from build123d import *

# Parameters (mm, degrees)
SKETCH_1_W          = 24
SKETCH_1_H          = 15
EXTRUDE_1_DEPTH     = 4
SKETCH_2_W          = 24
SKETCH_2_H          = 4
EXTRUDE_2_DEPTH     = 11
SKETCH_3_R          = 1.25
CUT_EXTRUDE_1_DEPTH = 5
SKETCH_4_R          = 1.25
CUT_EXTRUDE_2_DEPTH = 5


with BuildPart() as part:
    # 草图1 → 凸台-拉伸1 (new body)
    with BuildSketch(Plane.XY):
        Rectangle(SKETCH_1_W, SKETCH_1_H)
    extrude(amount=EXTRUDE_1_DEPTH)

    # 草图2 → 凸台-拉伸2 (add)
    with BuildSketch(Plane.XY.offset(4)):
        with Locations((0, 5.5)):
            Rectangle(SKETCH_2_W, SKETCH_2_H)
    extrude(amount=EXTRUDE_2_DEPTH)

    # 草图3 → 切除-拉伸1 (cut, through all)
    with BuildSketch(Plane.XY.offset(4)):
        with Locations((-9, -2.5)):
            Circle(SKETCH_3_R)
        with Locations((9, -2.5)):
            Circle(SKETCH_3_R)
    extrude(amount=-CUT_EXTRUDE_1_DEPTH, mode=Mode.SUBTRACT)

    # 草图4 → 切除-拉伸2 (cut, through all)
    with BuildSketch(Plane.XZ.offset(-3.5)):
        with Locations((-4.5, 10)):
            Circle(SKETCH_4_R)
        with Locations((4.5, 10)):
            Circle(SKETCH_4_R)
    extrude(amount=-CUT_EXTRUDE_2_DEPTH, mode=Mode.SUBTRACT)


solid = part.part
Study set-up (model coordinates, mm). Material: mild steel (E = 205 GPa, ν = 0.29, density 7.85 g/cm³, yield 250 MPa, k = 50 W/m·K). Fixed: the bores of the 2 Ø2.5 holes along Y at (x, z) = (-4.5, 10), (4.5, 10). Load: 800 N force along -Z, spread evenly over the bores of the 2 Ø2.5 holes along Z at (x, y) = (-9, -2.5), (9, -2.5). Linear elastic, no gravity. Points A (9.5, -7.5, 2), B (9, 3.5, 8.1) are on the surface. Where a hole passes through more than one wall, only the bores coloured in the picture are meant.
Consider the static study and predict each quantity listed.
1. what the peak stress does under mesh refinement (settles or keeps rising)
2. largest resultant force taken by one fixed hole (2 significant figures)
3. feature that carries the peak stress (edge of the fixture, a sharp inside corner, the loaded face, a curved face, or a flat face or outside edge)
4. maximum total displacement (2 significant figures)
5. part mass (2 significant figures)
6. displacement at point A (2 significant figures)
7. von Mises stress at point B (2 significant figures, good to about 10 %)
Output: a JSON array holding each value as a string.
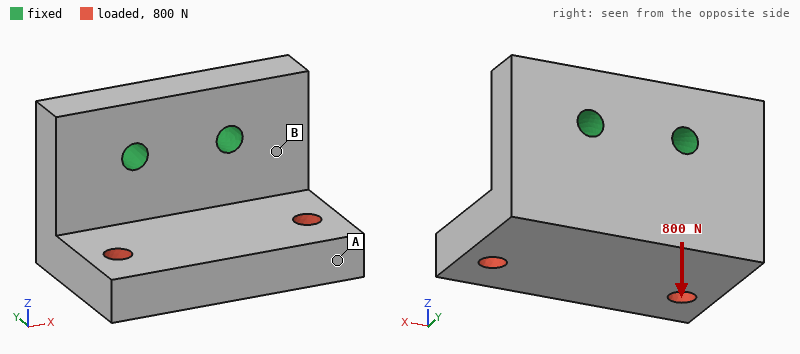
["keeps rising", "400 N", "edge of the fixture", "37 µm", "19 g", "34 µm", "74 MPa"]
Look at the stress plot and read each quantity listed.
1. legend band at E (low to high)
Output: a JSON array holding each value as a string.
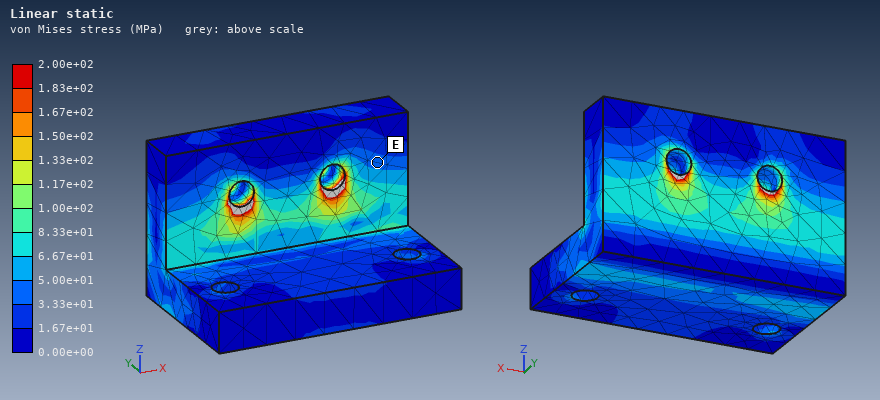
["3.33e+01 to 5.00e+01 MPa"]
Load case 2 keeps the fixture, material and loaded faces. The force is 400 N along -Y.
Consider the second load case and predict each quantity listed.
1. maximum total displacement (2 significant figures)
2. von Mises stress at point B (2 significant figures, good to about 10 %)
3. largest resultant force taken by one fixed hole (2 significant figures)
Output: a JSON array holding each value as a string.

["8.7 µm", "22 MPa", "200 N"]
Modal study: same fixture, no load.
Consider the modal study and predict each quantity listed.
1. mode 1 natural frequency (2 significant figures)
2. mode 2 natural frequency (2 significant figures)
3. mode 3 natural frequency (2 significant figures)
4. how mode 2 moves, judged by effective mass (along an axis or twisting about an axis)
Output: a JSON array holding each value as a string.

["9500 Hz", "14 kHz", "23 kHz", "along X"]
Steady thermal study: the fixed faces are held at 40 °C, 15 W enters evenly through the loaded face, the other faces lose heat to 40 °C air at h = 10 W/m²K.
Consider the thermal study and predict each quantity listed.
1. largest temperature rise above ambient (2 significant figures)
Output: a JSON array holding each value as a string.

["57 K"]
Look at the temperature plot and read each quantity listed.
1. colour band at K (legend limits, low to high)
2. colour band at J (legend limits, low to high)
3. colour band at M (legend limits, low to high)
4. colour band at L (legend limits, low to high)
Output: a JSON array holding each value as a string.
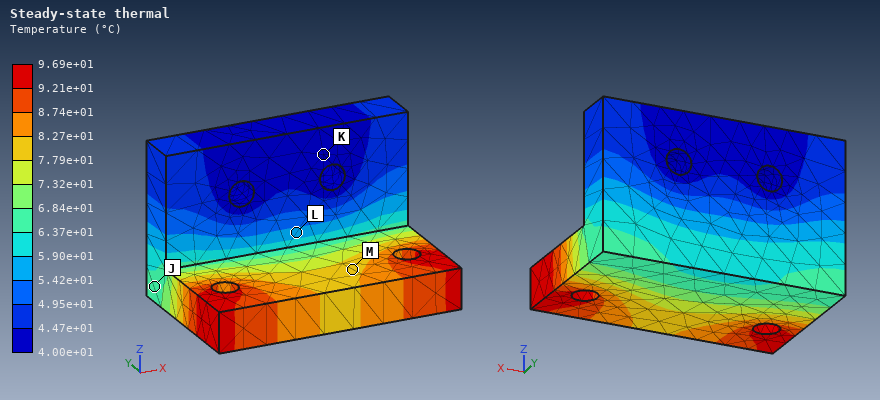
["4.00e+01 to 4.47e+01 °C", "6.37e+01 to 6.84e+01 °C", "7.79e+01 to 8.27e+01 °C", "5.42e+01 to 5.90e+01 °C"]
